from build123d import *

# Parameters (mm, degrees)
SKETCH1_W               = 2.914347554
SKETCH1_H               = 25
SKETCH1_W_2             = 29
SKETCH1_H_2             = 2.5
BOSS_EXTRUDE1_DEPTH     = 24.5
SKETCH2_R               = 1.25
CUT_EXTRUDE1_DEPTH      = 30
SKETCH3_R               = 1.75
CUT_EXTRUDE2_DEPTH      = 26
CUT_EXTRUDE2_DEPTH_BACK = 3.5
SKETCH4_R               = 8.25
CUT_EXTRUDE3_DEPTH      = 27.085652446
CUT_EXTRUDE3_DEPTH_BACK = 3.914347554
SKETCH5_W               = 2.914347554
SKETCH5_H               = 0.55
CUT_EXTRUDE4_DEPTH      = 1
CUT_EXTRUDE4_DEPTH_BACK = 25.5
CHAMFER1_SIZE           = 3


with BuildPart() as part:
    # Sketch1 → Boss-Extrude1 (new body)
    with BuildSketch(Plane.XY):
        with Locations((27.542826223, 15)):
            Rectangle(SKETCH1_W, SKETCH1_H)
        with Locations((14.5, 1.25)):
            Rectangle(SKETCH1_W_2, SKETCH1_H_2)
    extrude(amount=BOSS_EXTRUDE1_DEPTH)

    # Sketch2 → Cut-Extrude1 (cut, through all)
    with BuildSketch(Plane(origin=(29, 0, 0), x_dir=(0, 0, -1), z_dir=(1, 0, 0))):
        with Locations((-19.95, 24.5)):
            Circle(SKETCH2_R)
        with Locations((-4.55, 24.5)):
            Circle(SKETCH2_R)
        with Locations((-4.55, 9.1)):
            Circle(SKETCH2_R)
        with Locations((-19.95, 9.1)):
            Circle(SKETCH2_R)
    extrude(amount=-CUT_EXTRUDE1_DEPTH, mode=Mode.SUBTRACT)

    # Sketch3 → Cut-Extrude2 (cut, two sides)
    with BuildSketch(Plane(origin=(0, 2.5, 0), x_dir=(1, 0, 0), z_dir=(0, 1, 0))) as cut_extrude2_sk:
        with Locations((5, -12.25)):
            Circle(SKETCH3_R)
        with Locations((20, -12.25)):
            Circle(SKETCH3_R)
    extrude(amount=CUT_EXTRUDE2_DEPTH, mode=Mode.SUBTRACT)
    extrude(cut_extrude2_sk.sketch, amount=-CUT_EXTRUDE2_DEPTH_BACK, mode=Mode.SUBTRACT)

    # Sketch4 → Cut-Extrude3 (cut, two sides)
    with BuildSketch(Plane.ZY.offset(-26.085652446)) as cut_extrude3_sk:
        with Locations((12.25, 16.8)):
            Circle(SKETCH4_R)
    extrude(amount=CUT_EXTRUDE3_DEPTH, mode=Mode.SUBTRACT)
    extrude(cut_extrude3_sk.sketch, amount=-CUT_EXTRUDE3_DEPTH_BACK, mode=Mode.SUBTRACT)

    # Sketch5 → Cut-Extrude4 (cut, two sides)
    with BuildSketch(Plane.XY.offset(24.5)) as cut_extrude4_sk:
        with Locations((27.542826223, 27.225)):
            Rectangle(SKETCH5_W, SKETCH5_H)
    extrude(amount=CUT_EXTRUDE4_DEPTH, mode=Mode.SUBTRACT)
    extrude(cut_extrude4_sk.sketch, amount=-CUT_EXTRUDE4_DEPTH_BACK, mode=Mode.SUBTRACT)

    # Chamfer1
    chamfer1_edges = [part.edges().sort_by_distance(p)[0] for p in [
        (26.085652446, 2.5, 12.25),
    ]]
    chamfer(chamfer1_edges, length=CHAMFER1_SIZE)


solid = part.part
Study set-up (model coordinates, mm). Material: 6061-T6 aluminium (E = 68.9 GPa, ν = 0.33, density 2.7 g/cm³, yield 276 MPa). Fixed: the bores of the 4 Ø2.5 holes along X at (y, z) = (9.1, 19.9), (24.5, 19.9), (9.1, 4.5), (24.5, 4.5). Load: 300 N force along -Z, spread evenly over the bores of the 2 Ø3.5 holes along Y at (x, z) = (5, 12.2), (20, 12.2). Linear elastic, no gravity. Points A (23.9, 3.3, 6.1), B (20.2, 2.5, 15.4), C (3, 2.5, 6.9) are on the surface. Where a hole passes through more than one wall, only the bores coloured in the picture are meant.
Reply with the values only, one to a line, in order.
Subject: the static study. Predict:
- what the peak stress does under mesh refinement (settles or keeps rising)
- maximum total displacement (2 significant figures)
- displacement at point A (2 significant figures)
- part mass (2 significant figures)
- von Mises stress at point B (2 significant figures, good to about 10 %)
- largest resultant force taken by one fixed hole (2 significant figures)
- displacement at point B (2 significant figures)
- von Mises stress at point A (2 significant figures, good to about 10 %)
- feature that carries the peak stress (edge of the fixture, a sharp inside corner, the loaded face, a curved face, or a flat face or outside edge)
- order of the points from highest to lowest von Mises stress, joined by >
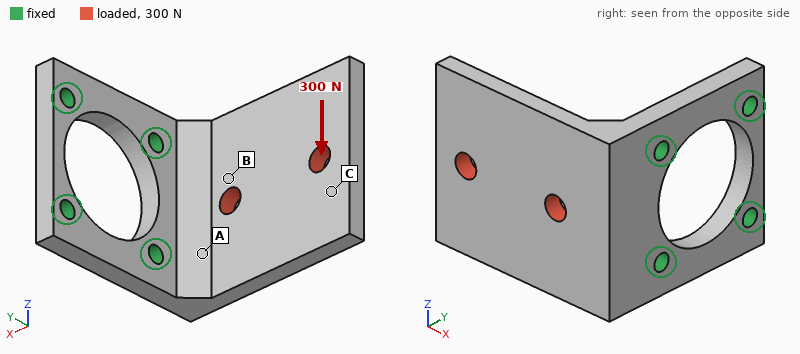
keeps rising
51 µm
8.9 µm
7.8 g
24 MPa
320 N
13 µm
37 MPa
edge of the fixture
A > B > C
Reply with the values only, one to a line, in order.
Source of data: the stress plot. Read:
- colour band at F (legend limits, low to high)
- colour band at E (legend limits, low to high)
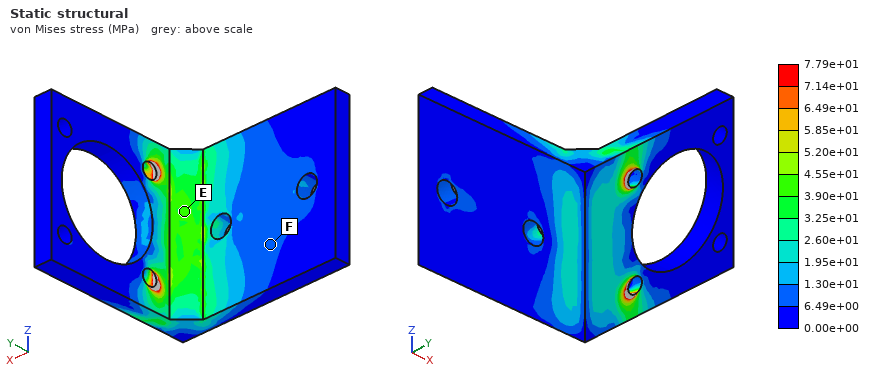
6.49e+00 to 1.30e+01 MPa
3.90e+01 to 4.55e+01 MPa
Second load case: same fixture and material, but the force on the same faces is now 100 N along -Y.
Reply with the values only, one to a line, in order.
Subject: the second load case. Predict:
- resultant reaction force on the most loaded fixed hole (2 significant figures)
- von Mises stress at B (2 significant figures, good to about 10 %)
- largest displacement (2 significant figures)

63 N
36 MPa
0.17 mm
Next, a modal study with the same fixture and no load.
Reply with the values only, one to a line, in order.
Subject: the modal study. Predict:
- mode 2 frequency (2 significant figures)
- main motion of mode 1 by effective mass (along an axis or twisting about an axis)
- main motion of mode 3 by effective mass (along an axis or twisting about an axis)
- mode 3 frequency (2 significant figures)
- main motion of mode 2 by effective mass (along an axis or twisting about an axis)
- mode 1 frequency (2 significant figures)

6300 Hz
along Y
along Z
8700 Hz
along Z
2400 Hz
